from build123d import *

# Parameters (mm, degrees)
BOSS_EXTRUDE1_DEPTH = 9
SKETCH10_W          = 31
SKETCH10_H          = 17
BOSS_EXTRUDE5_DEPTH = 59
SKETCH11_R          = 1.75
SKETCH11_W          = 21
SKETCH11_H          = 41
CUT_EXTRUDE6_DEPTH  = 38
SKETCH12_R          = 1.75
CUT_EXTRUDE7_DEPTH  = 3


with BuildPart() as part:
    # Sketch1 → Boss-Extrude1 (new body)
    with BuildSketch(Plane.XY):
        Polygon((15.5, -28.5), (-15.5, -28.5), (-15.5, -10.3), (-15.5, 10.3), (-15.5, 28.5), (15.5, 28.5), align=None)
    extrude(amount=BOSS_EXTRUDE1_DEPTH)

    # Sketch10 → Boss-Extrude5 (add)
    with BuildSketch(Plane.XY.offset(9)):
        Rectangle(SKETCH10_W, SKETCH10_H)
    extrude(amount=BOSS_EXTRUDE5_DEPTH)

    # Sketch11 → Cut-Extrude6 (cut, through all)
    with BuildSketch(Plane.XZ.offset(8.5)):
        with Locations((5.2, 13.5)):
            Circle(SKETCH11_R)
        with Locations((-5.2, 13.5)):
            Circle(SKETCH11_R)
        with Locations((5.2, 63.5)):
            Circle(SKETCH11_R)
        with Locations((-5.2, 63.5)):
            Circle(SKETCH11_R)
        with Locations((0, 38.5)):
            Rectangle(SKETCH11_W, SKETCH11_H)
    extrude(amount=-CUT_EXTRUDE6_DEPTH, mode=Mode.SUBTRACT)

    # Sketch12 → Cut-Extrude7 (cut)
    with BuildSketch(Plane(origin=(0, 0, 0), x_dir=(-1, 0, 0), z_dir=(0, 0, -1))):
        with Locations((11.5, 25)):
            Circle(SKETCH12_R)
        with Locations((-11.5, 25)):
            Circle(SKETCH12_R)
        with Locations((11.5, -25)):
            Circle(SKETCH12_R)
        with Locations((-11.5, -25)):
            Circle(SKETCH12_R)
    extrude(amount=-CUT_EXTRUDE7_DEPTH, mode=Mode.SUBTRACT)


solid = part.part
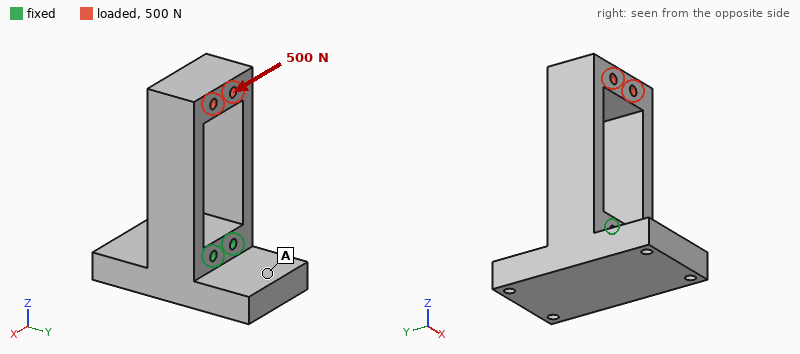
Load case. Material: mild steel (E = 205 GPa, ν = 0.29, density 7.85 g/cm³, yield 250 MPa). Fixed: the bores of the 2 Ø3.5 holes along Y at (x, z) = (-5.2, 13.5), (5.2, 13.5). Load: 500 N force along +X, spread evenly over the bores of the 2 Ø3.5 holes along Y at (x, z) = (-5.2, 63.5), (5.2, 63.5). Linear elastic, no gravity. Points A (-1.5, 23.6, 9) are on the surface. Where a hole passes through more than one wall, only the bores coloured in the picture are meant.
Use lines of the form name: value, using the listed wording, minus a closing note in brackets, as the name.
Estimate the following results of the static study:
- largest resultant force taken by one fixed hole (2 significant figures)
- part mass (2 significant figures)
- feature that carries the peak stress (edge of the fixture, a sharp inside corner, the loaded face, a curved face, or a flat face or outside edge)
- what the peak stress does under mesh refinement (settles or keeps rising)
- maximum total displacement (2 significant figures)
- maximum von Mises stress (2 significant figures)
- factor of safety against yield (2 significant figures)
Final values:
largest resultant force taken by one fixed hole: 1.6 kN
part mass: 250 g
feature that carries the peak stress: a flat face or outside edge
what the peak stress does under mesh refinement: settles
maximum total displacement: 69 µm
maximum von Mises stress: 71 MPa
factor of safety against yield: 3.5
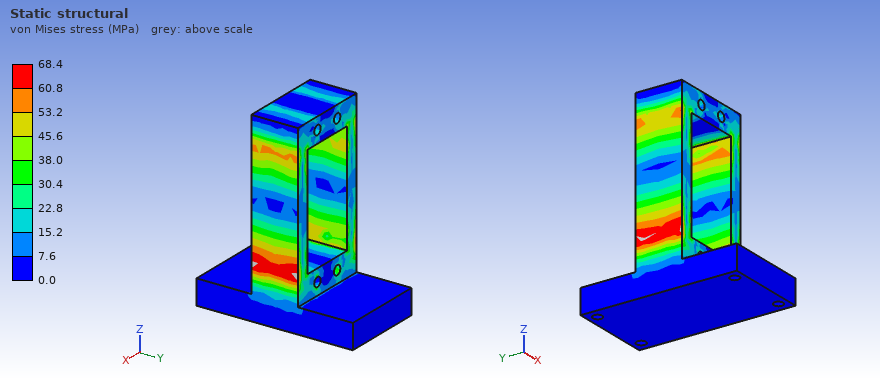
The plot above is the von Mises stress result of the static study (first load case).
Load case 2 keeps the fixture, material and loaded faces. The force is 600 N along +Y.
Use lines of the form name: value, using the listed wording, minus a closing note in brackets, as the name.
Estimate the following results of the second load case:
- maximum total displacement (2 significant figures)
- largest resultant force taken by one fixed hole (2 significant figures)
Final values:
maximum total displacement: 45 µm
largest resultant force taken by one fixed hole: 300 N
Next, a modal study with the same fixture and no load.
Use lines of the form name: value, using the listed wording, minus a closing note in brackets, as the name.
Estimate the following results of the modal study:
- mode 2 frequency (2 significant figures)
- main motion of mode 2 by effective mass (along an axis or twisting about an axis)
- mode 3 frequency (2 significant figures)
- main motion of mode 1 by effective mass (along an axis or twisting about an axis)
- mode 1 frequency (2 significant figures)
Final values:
mode 2 frequency: 2800 Hz
main motion of mode 2 by effective mass: along Y
mode 3 frequency: 5400 Hz
main motion of mode 1 by effective mass: along X
mode 1 frequency: 1900 Hz
